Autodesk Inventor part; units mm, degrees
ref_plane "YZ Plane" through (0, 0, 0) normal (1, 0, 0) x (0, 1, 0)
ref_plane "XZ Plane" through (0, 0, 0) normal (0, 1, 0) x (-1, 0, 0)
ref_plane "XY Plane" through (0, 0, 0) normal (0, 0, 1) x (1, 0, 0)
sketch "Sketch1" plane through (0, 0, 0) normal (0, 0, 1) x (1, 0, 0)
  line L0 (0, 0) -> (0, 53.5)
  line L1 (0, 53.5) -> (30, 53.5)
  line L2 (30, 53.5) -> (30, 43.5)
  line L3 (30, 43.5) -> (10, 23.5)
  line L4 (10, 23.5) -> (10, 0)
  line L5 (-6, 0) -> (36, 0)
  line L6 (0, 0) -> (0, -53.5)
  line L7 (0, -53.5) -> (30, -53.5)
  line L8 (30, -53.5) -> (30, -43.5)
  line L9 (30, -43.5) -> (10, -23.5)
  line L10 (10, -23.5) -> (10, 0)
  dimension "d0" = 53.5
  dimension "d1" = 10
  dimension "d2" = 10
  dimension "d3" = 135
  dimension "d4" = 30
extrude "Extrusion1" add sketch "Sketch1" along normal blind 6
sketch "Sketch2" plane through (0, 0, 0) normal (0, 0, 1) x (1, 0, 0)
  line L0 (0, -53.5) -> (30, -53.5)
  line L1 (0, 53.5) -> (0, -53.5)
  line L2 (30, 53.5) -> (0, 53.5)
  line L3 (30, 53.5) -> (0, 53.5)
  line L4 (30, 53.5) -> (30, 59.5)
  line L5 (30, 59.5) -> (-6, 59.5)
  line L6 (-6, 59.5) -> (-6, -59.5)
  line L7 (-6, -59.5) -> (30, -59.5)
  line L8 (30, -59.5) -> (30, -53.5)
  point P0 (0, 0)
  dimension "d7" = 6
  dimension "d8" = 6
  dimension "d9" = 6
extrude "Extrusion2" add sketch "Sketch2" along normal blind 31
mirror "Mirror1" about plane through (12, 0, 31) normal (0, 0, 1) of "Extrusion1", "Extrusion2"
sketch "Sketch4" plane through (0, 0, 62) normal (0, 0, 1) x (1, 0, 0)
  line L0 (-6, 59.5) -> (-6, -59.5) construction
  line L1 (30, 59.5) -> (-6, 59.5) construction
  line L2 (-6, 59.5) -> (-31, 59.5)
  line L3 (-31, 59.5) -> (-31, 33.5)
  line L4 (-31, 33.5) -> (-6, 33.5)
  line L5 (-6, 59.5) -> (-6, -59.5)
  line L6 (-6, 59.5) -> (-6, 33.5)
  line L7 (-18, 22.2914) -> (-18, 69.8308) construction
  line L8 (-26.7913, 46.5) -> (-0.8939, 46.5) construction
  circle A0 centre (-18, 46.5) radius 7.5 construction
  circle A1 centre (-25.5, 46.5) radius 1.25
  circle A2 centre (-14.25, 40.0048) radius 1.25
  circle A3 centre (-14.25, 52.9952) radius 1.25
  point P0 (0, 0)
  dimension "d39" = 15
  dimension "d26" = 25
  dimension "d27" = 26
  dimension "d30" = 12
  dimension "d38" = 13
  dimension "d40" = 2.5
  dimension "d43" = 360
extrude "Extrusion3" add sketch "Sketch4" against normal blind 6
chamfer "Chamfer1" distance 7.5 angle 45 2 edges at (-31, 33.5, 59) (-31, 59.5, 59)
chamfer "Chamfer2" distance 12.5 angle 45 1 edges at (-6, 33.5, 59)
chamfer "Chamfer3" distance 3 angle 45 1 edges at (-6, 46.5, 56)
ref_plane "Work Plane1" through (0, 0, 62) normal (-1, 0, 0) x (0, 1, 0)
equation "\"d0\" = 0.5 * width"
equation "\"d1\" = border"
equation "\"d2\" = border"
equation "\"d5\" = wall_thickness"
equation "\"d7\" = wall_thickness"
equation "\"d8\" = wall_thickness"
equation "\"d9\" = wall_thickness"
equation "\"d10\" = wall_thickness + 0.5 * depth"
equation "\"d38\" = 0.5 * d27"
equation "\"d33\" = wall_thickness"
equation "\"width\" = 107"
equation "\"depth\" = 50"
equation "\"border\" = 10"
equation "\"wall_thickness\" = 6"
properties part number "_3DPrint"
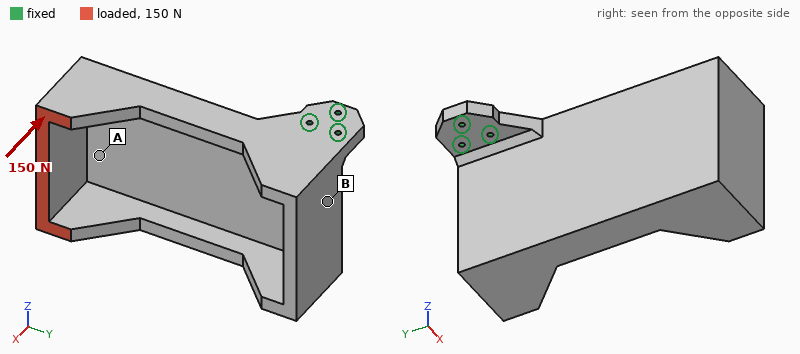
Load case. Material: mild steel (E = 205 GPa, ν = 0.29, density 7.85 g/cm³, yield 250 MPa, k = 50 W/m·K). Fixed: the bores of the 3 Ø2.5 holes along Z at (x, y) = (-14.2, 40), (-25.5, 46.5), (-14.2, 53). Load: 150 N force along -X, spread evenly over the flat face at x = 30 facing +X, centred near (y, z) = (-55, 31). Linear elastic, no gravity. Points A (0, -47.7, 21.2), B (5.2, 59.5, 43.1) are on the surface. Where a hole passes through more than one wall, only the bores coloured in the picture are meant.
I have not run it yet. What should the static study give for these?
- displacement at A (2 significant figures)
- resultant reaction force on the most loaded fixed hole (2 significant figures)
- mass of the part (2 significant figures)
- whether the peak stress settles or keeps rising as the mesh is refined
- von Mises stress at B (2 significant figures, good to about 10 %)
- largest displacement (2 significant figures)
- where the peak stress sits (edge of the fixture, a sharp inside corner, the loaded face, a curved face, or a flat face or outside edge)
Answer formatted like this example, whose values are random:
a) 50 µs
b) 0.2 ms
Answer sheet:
a) 67 µm
b) 830 N
c) 730 g
d) keeps rising
e) 6.2 MPa
f) 98 µm
g) edge of the fixture
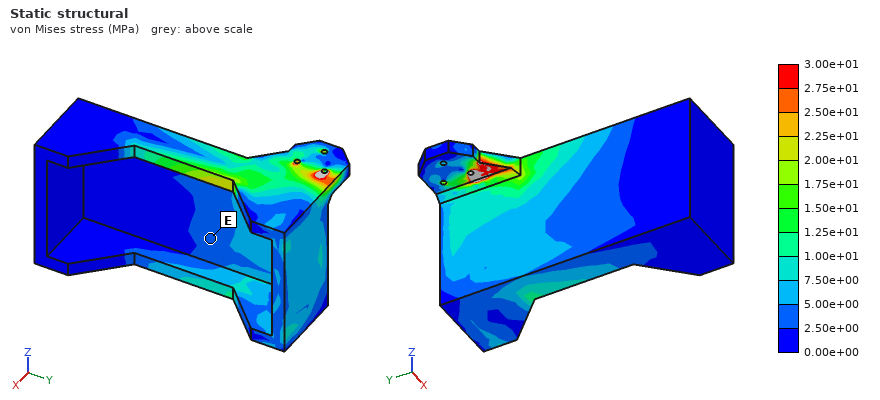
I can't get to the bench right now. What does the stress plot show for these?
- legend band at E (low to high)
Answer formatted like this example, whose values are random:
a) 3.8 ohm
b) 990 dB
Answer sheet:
a) 2.50e+00 to 5.00e+00 MPa
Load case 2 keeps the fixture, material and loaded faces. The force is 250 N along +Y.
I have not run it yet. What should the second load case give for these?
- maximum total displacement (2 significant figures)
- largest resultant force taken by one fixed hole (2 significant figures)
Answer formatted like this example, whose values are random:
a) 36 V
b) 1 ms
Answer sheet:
a) 49 µm
b) 760 N
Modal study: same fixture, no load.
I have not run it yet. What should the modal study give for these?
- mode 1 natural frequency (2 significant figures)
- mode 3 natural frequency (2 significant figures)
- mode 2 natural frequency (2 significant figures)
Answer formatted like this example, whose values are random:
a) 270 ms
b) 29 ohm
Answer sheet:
a) 380 Hz
b) 820 Hz
c) 530 Hz
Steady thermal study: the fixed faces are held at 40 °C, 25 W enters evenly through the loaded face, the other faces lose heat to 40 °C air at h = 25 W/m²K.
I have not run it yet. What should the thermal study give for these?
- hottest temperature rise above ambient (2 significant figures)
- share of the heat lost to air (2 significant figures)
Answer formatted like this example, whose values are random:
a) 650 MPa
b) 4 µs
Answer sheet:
a) 67 K
b) 80 %
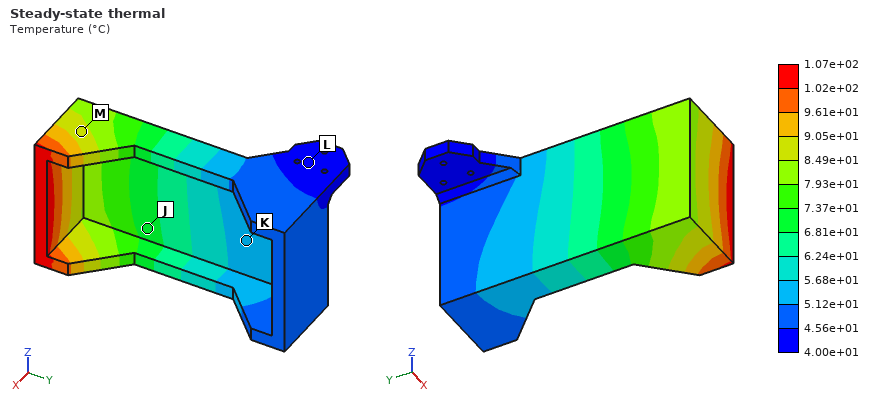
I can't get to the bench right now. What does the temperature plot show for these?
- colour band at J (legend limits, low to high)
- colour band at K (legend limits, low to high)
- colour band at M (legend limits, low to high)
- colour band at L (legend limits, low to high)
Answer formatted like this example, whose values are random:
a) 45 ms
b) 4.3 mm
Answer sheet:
a) 6.81e+01 to 7.37e+01 °C
b) 5.12e+01 to 5.68e+01 °C
c) 8.49e+01 to 9.05e+01 °C
d) 4.00e+01 to 4.56e+01 °C
